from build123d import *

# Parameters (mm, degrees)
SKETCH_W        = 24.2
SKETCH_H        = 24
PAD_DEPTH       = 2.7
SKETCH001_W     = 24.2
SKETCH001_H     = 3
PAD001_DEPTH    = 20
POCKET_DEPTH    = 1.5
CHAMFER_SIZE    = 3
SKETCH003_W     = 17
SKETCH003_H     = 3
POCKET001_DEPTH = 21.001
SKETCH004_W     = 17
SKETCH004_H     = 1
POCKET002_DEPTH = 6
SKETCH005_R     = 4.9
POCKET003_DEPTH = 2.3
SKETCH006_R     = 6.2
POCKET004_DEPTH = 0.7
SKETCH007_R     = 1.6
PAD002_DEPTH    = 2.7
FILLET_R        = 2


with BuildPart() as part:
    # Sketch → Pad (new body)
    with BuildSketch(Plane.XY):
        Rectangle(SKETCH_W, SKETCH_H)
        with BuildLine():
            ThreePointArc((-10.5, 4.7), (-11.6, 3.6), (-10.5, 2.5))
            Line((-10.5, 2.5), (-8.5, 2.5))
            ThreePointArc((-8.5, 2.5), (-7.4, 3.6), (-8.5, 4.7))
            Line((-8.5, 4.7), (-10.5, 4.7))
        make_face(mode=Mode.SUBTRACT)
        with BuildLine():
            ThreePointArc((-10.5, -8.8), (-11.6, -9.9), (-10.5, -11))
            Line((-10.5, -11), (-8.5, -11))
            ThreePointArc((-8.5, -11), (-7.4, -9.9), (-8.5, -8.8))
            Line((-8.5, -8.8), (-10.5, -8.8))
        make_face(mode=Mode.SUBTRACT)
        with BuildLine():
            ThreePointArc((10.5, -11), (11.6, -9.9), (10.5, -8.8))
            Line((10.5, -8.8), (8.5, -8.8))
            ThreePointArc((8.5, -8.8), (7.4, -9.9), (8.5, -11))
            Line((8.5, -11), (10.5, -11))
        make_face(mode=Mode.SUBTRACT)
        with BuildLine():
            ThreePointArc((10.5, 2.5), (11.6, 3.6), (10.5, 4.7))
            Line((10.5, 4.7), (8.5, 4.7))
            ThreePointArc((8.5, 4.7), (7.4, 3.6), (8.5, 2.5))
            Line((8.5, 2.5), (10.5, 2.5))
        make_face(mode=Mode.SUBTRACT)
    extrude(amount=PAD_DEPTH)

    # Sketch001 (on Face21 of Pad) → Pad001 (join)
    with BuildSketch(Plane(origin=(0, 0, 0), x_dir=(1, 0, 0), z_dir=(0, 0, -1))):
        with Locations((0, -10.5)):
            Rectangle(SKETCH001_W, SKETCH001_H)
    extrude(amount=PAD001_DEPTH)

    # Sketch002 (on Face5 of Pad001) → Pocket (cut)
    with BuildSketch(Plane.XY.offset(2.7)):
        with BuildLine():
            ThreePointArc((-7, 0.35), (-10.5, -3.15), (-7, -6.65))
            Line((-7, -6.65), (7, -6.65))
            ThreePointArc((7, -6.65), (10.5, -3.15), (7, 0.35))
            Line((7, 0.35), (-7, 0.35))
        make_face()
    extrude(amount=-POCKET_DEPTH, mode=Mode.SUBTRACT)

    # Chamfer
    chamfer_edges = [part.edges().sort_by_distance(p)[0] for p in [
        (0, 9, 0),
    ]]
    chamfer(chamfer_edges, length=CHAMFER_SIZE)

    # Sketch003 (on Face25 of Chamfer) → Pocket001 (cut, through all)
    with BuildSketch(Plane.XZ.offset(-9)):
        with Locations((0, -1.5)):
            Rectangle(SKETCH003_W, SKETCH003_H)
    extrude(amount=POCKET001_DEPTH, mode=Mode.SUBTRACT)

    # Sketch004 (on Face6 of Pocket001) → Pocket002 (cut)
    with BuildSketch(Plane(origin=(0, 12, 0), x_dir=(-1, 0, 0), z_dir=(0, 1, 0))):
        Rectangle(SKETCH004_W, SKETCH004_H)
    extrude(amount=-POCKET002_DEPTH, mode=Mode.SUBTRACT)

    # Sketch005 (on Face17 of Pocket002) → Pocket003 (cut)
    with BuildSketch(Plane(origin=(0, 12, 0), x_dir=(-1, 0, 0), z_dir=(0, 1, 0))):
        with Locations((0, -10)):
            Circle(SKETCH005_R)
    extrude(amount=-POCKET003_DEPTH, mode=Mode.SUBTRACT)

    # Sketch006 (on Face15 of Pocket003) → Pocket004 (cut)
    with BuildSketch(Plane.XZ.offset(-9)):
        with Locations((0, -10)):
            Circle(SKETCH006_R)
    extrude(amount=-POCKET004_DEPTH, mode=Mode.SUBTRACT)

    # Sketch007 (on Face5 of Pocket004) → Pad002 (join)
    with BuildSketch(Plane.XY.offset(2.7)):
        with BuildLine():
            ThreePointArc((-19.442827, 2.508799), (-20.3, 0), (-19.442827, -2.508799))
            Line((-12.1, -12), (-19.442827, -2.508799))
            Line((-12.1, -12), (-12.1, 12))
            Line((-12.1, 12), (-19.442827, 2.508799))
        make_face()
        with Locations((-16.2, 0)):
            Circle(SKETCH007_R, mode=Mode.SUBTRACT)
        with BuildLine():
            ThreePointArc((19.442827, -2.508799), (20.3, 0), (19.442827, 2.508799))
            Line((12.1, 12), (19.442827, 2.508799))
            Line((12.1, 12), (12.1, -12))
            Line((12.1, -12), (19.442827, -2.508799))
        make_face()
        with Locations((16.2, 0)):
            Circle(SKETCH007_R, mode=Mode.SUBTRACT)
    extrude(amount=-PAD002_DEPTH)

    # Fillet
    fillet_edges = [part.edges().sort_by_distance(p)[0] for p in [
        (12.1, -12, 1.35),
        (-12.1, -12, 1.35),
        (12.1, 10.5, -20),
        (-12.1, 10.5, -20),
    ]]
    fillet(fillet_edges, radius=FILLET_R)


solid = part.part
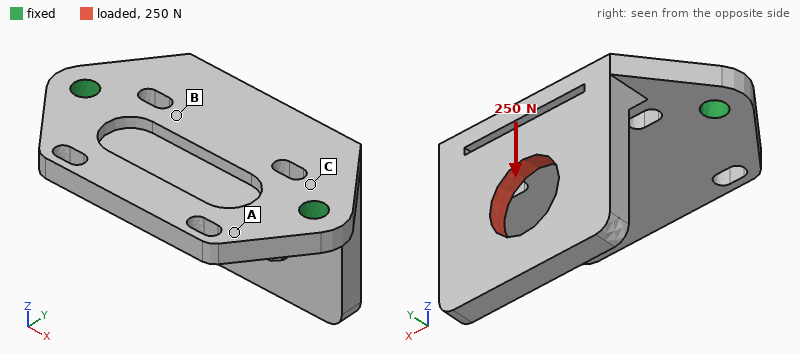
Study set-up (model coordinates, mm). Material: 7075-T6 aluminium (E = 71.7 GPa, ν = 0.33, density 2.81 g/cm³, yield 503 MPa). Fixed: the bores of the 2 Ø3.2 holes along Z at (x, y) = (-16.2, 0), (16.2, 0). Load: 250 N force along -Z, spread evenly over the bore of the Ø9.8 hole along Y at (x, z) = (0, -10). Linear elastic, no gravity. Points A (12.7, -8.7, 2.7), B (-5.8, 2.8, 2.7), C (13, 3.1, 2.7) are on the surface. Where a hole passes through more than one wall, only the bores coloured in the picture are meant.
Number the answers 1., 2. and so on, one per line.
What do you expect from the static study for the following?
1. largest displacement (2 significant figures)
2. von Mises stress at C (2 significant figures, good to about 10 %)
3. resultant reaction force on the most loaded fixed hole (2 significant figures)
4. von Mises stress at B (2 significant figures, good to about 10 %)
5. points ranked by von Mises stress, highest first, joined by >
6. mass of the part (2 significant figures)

1. 0.15 mm
2. 83 MPa
3. 130 N
4. 25 MPa
5. C > B > A
6. 8.3 g
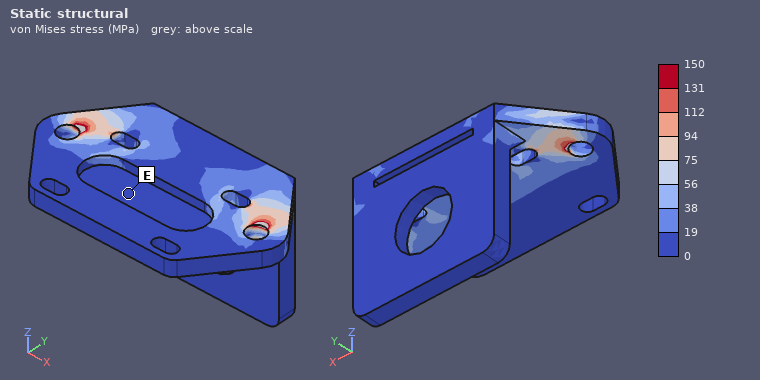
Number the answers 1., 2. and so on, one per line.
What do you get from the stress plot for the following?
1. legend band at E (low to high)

1. 0 to 19 MPa
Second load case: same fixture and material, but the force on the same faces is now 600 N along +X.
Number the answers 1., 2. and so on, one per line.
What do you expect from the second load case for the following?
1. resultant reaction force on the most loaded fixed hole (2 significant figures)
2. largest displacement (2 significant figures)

1. 430 N
2. 98 µm
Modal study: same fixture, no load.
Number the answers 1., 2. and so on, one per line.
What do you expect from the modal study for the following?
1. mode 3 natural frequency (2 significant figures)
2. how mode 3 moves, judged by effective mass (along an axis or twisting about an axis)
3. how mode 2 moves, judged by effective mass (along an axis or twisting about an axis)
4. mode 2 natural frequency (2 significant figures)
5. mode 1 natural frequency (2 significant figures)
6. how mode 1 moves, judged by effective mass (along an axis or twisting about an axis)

1. 8200 Hz
2. along Z
3. along X
4. 6800 Hz
5. 2600 Hz
6. along Y
